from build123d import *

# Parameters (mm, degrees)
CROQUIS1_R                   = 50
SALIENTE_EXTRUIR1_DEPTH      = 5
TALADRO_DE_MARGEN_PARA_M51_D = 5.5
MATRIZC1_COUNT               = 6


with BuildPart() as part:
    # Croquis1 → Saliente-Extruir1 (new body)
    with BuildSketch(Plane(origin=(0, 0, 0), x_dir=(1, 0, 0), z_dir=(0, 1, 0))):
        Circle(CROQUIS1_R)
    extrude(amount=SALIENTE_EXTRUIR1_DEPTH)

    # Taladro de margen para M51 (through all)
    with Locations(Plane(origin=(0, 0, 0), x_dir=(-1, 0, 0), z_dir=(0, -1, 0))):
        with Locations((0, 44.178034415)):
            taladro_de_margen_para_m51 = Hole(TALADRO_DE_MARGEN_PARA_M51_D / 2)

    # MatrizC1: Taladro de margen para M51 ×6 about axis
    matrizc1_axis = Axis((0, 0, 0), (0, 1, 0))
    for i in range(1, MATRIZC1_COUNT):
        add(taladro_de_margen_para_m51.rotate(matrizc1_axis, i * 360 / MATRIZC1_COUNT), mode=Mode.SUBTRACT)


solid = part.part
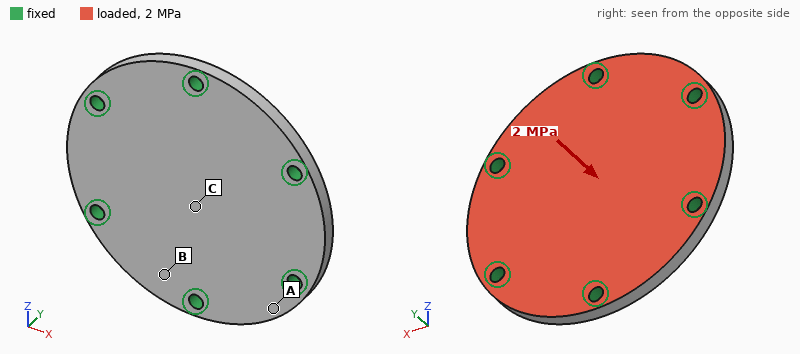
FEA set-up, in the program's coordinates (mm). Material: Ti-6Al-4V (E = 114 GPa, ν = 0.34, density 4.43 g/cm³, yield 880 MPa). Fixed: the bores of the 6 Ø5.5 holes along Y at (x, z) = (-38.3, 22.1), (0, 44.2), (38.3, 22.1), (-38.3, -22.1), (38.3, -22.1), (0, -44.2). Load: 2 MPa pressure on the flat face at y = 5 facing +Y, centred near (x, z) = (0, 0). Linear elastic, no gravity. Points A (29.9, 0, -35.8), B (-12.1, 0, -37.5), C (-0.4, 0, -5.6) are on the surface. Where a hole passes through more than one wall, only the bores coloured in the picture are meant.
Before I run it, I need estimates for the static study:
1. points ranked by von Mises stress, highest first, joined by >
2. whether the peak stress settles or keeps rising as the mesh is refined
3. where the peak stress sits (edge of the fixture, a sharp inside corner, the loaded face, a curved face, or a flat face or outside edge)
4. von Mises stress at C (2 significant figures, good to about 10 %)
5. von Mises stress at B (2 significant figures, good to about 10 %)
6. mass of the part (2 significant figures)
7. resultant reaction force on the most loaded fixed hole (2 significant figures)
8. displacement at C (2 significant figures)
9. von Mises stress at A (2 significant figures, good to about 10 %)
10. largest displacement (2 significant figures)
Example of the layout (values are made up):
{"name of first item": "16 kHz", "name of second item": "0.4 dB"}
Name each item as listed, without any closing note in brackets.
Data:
{"points ranked by von Mises stress, highest first, joined by >": "C > B > A", "whether the peak stress settles or keeps rising as the mesh is refined": "keeps rising", "where the peak stress sits": "edge of the fixture", "von Mises stress at C": "84 MPa", "von Mises stress at B": "49 MPa", "mass of the part": "170 g", "resultant reaction force on the most loaded fixed hole": "2.6 kN", "displacement at C": "0.12 mm", "von Mises stress at A": "25 MPa", "largest displacement": "0.12 mm"}
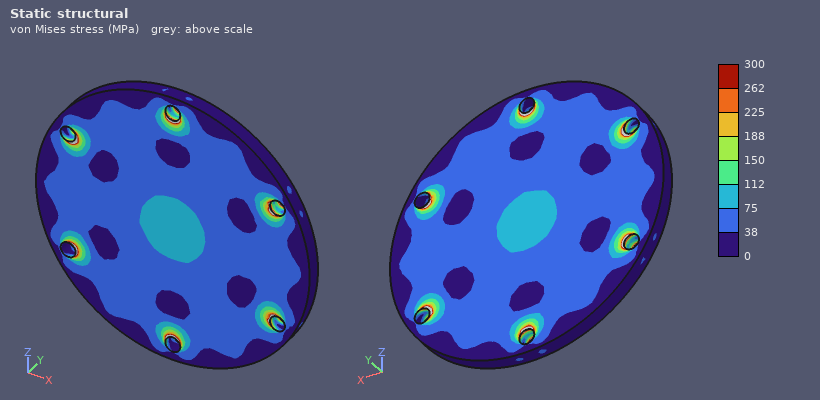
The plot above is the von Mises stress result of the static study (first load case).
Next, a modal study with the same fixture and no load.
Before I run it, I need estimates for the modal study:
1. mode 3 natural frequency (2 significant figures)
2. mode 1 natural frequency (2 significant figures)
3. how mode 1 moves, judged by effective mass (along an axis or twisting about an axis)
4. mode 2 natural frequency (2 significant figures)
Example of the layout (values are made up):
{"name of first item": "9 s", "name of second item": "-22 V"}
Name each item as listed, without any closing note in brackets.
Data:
{"mode 3 natural frequency": "11 kHz", "mode 1 natural frequency": "5400 Hz", "how mode 1 moves, judged by effective mass": "along Y", "mode 2 natural frequency": "11 kHz"}
